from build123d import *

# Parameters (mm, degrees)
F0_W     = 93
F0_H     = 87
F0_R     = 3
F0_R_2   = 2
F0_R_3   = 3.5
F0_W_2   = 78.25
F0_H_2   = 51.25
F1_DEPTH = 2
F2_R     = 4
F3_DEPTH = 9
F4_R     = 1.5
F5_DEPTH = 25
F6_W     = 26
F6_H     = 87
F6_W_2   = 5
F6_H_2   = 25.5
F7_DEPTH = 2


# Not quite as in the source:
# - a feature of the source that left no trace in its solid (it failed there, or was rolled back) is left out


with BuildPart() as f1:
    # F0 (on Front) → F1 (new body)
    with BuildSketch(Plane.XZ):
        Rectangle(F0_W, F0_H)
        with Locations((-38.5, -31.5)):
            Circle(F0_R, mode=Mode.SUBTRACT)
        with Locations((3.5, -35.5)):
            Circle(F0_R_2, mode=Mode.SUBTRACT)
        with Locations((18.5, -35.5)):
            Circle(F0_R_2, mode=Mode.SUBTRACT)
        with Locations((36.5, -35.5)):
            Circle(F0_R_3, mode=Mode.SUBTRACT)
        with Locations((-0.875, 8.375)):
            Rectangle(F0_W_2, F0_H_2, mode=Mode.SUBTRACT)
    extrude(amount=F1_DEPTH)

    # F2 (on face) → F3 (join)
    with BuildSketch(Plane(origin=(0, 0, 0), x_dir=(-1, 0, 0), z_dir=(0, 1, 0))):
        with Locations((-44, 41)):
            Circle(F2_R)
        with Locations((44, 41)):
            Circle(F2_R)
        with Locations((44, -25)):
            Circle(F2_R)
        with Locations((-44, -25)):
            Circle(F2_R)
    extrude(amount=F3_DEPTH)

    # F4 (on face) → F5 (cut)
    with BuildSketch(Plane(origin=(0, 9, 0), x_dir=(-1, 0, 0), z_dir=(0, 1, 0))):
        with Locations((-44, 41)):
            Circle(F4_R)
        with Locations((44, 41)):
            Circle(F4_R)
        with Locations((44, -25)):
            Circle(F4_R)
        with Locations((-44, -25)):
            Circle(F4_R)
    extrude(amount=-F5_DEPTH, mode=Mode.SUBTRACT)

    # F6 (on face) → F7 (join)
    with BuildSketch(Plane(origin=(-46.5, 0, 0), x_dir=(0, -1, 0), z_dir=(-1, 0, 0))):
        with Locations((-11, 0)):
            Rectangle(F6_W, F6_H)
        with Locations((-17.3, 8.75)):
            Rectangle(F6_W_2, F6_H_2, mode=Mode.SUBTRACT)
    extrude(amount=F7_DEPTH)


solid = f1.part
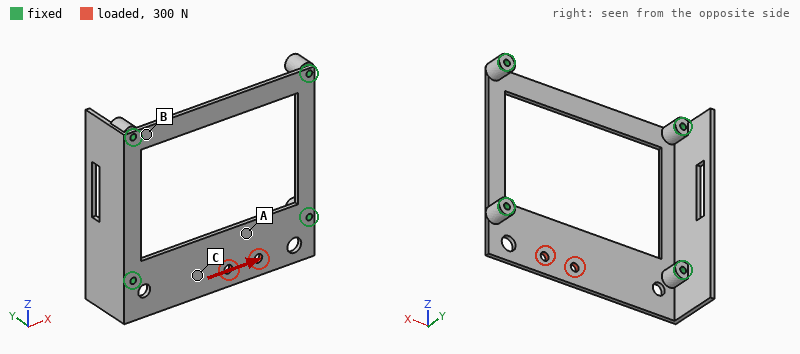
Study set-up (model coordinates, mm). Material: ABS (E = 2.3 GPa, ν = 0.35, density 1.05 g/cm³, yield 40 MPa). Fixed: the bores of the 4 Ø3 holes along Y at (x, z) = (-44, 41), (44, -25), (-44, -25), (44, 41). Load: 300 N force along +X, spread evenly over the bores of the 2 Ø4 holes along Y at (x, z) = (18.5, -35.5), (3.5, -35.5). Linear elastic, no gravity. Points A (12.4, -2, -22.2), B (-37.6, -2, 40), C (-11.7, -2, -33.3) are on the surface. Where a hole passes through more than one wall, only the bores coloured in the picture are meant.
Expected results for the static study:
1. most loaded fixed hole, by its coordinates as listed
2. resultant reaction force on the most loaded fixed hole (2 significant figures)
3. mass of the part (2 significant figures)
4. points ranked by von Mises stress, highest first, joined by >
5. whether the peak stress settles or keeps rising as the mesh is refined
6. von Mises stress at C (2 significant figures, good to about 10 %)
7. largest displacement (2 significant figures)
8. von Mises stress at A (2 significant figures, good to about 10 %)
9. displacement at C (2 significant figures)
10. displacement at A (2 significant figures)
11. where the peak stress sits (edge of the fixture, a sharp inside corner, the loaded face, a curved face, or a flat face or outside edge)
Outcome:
(44, -25)
170 N
14 g
C > A > B
keeps rising
3.5 MPa
0.11 mm
1.8 MPa
0.063 mm
0.063 mm
edge of the fixture
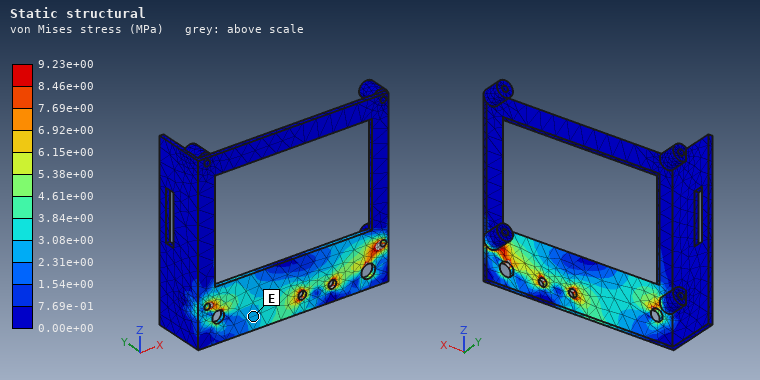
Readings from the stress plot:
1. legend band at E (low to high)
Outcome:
2.31e+00 to 3.08e+00 MPa
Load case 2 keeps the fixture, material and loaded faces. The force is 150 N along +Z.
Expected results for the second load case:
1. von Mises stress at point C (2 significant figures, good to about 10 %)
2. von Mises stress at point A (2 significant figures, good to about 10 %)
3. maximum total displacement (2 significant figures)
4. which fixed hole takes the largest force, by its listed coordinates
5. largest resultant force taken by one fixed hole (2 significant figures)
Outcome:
3.3 MPa
3.5 MPa
0.24 mm
(44, -25)
100 N
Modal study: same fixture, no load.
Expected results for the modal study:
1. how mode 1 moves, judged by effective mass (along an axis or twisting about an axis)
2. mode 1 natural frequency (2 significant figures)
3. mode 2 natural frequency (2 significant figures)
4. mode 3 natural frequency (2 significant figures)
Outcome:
along Y
380 Hz
440 Hz
800 Hz
